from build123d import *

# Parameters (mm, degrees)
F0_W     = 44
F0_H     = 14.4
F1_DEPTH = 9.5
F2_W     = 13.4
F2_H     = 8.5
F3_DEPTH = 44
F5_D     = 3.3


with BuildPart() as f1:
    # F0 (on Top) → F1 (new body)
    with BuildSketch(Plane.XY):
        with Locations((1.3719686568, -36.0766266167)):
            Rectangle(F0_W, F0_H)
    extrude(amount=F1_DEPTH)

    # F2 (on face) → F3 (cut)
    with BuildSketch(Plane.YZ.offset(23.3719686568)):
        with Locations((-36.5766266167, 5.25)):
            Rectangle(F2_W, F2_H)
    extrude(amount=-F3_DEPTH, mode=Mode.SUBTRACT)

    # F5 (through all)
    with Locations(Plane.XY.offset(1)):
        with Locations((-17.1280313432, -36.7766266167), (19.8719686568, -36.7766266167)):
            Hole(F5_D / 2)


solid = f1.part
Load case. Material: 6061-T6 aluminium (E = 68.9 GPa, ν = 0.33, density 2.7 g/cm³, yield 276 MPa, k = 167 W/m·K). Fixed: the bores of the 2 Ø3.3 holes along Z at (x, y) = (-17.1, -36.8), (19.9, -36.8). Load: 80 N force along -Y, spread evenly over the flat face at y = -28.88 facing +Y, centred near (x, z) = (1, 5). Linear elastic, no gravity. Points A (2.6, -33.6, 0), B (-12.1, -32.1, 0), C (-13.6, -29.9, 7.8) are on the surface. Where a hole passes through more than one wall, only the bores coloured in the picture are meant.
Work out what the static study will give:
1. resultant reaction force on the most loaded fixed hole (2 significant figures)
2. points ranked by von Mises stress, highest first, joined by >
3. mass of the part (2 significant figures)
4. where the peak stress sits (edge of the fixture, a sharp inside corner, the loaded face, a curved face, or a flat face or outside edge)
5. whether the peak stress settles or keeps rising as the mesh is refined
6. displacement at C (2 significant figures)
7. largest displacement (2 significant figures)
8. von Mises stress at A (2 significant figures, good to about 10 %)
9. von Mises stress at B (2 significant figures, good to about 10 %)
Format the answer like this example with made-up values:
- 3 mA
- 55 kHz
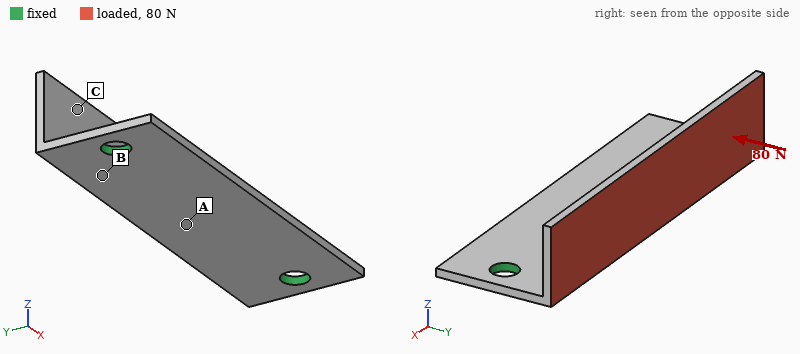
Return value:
- 40 N
- B > A > C
- 2.7 g
- edge of the fixture
- keeps rising
- 0.10 mm
- 0.14 mm
- 24 MPa
- 44 MPa
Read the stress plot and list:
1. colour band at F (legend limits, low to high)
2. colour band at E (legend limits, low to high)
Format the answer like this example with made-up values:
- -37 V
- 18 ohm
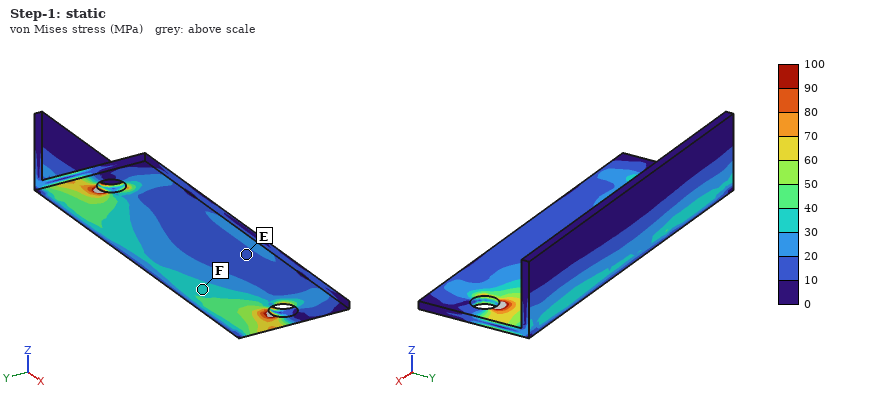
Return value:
- 30 to 40 MPa
- 10 to 20 MPa
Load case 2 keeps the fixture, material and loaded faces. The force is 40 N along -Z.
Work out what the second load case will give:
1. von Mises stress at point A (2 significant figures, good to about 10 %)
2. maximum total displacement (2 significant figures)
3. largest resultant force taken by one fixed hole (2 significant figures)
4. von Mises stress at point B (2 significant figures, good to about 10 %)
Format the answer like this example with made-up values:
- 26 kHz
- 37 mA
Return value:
- 6.5 MPa
- 64 µm
- 21 N
- 19 MPa
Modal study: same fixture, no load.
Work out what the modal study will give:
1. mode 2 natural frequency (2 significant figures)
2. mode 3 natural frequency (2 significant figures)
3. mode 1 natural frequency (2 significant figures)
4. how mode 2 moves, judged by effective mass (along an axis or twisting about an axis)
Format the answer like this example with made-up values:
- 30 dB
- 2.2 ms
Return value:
- 5500 Hz
- 5800 Hz
- 3700 Hz
- along Z
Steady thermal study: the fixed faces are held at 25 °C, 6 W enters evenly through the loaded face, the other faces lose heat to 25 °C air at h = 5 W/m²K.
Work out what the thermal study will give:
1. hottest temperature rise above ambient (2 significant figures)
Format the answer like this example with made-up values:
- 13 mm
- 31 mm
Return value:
- 15 K
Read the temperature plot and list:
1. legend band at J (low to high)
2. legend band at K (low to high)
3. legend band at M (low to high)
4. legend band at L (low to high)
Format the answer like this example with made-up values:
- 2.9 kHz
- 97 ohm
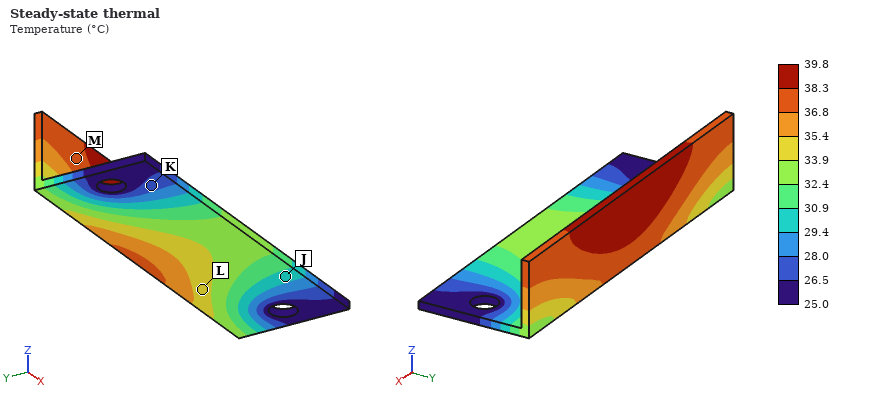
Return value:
- 29.4 to 30.9 °C
- 26.5 to 28.0 °C
- 36.8 to 38.3 °C
- 33.9 to 35.4 °C
